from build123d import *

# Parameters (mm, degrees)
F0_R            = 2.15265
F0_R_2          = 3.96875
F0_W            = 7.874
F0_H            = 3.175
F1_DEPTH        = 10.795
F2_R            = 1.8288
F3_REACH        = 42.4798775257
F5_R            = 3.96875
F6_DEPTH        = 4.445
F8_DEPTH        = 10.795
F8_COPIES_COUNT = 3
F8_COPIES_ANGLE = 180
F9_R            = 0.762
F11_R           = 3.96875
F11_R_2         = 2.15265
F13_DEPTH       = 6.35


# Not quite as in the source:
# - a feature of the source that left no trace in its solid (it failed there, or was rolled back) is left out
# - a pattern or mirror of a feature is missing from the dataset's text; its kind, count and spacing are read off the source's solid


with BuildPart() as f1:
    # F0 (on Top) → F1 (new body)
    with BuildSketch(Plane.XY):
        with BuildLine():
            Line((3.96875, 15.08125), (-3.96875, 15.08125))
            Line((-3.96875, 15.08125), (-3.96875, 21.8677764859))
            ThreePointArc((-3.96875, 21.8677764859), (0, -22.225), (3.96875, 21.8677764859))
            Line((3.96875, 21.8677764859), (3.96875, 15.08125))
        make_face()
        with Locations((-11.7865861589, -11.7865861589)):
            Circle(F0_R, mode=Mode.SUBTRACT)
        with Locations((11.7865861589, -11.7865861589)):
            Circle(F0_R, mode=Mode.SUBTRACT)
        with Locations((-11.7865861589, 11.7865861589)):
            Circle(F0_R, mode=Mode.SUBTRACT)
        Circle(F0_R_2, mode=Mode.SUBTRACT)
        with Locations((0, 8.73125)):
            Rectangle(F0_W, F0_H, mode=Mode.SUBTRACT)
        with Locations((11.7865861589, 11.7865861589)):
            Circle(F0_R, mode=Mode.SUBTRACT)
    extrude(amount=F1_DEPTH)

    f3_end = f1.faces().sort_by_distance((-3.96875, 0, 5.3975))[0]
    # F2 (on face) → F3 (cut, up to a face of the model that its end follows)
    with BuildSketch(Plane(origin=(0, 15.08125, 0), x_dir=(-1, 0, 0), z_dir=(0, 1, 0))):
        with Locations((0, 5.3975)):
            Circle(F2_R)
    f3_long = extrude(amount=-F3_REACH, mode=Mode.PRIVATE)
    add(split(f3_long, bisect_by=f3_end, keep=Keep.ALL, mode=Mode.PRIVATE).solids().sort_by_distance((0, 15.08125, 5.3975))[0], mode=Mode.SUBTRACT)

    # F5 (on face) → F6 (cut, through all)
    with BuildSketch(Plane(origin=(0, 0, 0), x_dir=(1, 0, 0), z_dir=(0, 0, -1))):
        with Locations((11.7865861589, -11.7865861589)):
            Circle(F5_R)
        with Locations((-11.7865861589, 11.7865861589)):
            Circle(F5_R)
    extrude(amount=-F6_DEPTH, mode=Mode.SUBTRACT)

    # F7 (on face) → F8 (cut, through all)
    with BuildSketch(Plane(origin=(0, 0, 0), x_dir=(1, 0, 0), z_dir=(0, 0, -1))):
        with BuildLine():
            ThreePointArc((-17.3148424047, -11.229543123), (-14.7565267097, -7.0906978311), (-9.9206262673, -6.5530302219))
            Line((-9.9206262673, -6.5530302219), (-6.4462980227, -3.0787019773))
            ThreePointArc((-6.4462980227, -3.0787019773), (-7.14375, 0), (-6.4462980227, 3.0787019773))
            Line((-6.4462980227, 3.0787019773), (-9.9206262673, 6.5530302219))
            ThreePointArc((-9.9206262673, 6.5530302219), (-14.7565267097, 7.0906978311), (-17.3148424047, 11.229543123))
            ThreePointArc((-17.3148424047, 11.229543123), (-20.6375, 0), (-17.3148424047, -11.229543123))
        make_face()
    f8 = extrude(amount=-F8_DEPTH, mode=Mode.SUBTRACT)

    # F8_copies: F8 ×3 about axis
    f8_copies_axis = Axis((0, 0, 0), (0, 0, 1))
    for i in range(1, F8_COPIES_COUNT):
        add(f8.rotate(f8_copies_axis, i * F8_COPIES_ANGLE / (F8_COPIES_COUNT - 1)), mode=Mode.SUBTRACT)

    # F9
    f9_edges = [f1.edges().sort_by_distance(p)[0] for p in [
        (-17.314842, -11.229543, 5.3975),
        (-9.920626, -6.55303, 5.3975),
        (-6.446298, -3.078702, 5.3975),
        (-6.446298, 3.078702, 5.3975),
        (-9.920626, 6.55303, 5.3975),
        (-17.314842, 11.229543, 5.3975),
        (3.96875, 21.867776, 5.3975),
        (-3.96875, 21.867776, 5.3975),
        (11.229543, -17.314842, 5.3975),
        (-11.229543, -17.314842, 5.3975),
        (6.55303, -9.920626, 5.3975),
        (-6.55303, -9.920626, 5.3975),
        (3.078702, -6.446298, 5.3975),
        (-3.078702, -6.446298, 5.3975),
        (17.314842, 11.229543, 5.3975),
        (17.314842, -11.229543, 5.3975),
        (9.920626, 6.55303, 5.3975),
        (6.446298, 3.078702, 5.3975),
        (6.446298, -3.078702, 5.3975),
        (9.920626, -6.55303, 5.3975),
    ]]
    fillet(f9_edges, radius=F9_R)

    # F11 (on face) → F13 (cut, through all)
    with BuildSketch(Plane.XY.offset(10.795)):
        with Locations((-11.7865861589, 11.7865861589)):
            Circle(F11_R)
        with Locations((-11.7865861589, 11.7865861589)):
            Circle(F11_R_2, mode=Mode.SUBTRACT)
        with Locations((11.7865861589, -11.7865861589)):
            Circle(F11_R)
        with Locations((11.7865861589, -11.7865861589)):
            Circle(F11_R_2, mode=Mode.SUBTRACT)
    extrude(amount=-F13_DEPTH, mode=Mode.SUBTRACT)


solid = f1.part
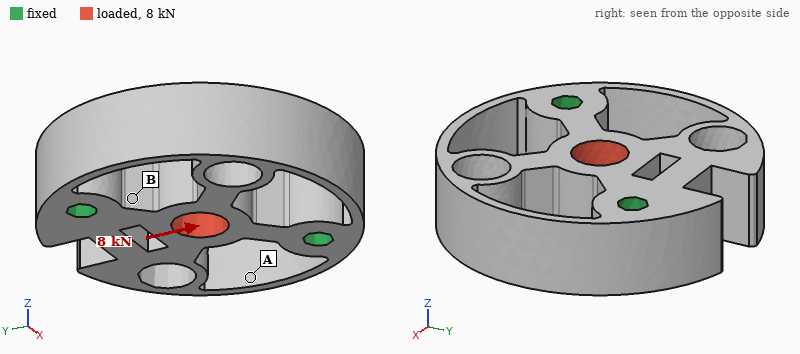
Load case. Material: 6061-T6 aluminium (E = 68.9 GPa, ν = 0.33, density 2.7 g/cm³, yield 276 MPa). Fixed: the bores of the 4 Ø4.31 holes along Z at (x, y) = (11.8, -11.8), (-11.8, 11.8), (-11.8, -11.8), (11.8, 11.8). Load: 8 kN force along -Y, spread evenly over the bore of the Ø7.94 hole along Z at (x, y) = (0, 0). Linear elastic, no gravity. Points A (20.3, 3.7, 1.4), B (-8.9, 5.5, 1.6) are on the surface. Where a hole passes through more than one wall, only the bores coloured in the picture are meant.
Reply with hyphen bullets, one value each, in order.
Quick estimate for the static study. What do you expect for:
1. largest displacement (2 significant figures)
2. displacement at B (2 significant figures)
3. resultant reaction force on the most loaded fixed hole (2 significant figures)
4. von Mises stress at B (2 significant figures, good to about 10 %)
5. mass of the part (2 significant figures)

- 20 µm
- 4.8 µm
- 2.5 kN
- 65 MPa
- 21 g
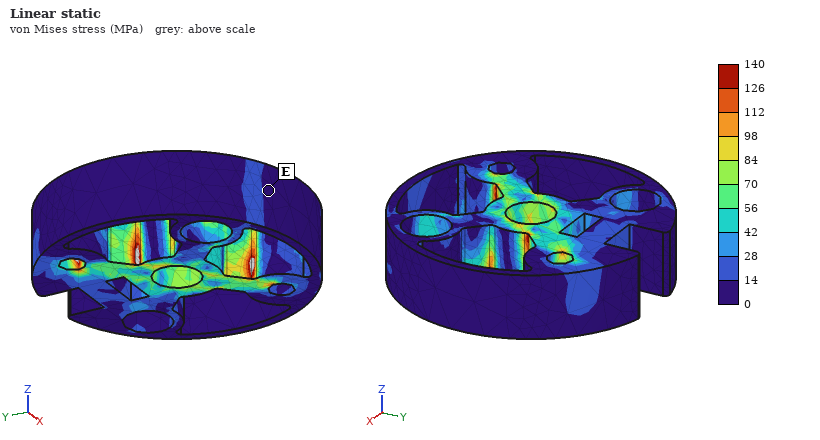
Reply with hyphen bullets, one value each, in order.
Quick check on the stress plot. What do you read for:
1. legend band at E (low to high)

- 0 to 14 MPa
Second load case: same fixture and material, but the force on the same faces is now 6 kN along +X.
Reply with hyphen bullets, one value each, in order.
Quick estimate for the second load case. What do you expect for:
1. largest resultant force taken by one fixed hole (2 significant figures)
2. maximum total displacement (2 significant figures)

- 1.9 kN
- 15 µm
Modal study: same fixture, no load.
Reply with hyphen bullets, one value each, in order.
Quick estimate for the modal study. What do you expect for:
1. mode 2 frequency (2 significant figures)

- 26 kHz
